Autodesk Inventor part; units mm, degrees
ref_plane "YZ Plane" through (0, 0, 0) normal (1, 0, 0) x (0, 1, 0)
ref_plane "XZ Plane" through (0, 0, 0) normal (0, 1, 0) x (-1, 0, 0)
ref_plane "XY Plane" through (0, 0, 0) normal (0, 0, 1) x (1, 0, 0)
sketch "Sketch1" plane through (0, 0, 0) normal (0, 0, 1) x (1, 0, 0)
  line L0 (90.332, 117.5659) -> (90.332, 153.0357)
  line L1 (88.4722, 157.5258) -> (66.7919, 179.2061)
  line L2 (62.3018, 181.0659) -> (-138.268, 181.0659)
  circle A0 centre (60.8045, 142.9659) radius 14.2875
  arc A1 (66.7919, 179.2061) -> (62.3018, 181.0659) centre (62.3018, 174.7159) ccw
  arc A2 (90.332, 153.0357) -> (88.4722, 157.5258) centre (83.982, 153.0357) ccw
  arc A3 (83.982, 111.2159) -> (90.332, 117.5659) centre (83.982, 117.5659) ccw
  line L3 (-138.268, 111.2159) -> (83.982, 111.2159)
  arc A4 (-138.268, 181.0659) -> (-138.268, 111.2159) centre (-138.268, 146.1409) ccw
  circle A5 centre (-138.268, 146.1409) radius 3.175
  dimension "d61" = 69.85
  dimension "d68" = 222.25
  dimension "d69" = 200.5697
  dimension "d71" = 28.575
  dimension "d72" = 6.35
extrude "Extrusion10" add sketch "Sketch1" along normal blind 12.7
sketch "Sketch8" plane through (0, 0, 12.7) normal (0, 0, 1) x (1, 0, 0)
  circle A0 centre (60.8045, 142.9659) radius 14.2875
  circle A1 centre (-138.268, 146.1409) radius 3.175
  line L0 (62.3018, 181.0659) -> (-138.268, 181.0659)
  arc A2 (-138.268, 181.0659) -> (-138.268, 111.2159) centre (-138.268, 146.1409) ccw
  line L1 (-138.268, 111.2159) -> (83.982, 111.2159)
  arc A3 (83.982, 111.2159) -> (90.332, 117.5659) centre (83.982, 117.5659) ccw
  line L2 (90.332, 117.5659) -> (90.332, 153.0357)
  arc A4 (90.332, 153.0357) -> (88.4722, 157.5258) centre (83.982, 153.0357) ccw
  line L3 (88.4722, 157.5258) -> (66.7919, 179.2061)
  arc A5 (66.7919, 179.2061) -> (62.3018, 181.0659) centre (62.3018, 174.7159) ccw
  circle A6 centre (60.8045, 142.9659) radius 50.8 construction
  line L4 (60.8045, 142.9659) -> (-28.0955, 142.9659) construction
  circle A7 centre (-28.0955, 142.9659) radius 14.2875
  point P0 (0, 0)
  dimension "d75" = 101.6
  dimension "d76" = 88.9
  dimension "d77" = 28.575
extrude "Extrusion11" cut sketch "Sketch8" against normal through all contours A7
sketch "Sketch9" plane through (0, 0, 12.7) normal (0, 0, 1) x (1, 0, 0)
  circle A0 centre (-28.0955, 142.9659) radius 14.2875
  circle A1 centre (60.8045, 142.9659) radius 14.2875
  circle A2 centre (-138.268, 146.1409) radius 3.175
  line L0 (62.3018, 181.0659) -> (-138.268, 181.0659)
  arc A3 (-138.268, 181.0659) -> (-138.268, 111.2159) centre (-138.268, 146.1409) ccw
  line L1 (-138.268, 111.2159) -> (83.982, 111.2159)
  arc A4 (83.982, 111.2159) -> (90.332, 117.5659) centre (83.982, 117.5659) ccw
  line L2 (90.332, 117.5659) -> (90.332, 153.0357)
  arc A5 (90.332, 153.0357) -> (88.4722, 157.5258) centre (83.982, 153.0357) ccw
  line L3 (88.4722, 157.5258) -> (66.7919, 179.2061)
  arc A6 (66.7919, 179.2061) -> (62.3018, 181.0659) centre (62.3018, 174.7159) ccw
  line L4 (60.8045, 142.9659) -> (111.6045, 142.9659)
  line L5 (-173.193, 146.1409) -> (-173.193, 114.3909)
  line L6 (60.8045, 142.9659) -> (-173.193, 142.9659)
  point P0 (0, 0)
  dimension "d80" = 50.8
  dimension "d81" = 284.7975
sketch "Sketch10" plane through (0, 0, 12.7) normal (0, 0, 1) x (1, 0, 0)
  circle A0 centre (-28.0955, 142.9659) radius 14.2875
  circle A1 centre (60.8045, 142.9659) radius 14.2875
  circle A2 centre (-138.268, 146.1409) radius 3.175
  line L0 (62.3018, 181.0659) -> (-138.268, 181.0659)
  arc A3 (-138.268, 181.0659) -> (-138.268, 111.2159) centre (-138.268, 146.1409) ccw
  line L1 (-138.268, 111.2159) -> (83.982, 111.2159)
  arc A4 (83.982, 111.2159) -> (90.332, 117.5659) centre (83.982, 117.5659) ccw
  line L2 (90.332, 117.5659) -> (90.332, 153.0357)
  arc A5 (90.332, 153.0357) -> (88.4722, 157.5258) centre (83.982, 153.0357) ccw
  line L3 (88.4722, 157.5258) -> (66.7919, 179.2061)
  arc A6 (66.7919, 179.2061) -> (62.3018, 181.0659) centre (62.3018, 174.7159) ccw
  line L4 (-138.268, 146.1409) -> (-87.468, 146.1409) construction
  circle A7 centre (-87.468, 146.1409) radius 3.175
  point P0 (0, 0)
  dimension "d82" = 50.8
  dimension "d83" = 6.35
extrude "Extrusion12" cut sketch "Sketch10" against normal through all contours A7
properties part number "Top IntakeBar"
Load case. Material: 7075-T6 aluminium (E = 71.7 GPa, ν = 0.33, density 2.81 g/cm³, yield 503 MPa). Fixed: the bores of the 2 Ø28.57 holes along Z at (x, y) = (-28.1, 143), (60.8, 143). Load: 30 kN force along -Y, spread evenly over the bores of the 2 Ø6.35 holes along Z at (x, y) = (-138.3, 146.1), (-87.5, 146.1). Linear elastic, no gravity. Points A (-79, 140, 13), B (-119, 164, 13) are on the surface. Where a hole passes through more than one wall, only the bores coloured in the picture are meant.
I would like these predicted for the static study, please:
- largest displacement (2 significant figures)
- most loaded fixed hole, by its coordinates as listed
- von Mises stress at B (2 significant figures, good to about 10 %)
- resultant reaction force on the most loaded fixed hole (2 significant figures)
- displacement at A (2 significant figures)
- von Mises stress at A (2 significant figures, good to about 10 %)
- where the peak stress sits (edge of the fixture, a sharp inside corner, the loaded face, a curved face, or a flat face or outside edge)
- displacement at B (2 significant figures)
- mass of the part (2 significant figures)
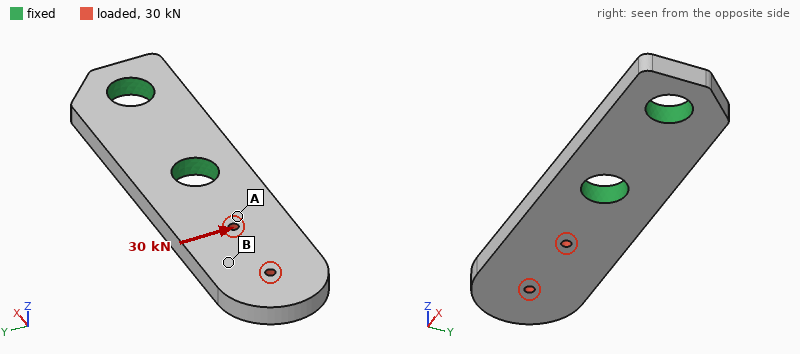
0.76 mm
(-28.1, 143)
37 MPa
39 kN
0.21 mm
81 MPa
edge of the fixture
0.46 mm
580 g
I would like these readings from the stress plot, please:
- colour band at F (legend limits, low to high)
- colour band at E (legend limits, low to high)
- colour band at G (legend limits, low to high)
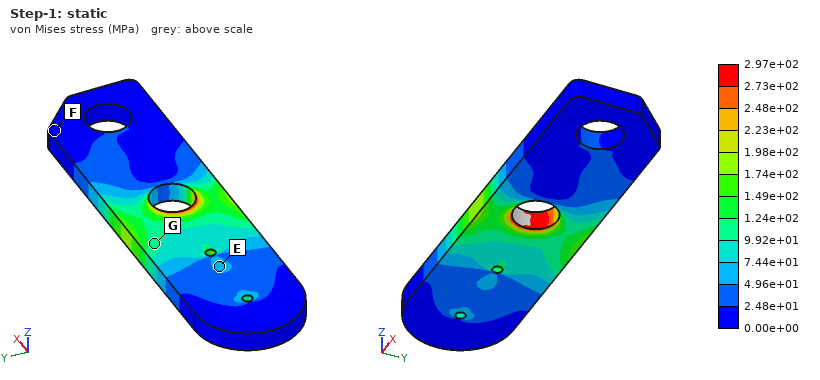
0.00e+00 to 2.48e+01 MPa
4.96e+01 to 7.44e+01 MPa
9.92e+01 to 1.24e+02 MPa
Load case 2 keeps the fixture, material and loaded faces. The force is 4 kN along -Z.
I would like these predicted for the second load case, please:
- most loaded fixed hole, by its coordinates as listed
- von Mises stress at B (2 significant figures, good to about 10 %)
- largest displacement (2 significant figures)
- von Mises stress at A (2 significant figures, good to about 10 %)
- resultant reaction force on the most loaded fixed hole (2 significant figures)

(-28.1, 143)
23 MPa
1.5 mm
67 MPa
4.0 kN
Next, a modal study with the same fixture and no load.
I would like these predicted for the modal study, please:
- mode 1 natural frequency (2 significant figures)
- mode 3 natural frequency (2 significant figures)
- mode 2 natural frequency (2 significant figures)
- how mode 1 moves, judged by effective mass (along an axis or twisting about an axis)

630 Hz
2300 Hz
2300 Hz
along Z
